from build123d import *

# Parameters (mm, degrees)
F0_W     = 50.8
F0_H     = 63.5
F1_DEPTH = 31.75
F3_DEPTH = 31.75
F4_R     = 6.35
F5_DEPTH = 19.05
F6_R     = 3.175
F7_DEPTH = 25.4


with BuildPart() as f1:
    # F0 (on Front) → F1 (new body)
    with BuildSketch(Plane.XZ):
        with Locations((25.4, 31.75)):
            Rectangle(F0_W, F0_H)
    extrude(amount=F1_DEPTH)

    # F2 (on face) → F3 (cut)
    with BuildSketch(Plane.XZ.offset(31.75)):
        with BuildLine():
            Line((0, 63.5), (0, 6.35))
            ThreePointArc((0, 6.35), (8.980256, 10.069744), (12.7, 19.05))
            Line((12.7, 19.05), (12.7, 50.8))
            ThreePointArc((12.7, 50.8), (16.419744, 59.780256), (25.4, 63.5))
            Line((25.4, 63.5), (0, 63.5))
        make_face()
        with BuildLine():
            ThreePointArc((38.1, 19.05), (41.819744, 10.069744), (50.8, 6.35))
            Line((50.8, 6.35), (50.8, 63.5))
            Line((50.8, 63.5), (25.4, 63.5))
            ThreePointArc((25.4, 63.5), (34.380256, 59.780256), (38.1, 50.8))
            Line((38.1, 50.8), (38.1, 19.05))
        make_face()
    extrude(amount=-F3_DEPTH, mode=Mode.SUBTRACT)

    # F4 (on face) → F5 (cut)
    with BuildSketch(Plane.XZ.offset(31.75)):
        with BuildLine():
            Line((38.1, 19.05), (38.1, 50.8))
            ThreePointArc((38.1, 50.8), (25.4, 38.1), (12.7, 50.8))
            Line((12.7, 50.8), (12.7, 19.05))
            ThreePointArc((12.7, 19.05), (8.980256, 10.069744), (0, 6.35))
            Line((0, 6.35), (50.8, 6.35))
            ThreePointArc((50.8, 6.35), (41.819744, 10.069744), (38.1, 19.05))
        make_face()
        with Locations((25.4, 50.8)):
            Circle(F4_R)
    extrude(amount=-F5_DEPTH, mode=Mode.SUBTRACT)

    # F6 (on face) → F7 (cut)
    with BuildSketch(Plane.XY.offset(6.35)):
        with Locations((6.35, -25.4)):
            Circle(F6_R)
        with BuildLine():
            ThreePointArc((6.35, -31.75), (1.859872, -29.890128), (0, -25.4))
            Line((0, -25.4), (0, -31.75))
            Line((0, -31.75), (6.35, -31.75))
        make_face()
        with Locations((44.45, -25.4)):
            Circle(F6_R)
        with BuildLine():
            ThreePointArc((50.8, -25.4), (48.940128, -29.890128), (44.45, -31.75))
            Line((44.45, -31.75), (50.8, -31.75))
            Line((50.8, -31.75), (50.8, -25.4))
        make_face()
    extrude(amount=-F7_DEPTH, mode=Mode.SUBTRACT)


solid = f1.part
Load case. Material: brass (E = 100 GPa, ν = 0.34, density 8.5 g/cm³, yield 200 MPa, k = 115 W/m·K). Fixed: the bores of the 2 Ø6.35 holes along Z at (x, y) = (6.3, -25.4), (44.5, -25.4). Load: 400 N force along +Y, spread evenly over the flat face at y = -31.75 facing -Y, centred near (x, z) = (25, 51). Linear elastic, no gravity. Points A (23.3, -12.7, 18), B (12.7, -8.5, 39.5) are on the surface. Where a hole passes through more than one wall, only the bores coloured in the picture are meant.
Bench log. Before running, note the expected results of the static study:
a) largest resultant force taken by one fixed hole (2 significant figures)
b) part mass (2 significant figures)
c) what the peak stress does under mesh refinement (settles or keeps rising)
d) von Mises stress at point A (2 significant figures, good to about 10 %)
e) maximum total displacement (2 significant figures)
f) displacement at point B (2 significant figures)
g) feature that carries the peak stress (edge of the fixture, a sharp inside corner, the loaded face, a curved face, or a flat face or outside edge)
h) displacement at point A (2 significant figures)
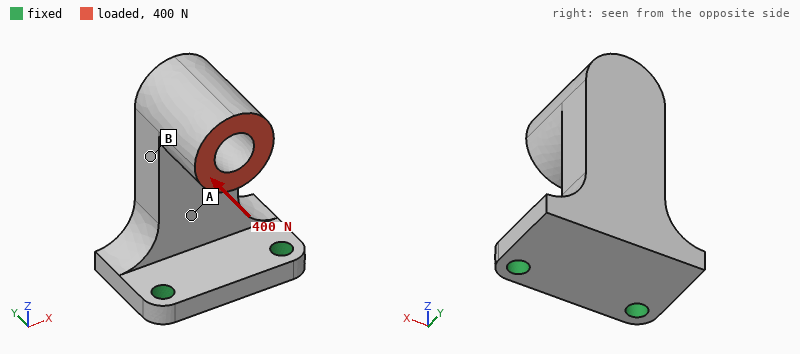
240 N
300 g
keeps rising
19 MPa
0.22 mm
0.12 mm
edge of the fixture
0.047 mm
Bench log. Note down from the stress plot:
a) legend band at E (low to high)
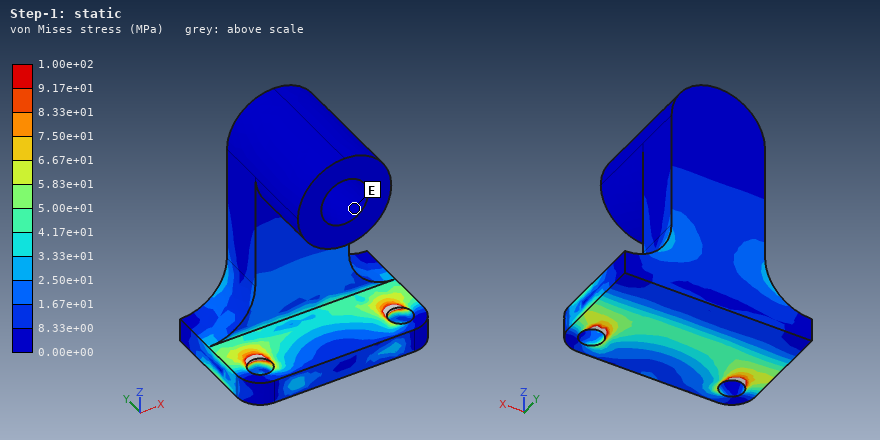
0.00e+00 to 8.33e+00 MPa
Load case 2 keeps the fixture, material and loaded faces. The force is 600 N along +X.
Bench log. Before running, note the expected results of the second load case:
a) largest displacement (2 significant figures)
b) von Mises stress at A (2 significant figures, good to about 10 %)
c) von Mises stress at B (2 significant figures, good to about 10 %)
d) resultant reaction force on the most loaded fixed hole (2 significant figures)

98 µm
31 MPa
18 MPa
830 N
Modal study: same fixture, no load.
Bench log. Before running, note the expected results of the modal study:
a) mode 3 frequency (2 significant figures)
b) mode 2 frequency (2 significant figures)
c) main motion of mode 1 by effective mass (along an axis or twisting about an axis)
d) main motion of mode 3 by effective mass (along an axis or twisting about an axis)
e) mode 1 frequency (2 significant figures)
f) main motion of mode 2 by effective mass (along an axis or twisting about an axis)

2900 Hz
1500 Hz
along Y
along Z
640 Hz
along X
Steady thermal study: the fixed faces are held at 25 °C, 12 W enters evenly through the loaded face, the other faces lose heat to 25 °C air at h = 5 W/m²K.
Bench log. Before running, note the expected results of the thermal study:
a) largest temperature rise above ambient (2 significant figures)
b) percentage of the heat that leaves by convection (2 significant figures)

24 K
4.9 %
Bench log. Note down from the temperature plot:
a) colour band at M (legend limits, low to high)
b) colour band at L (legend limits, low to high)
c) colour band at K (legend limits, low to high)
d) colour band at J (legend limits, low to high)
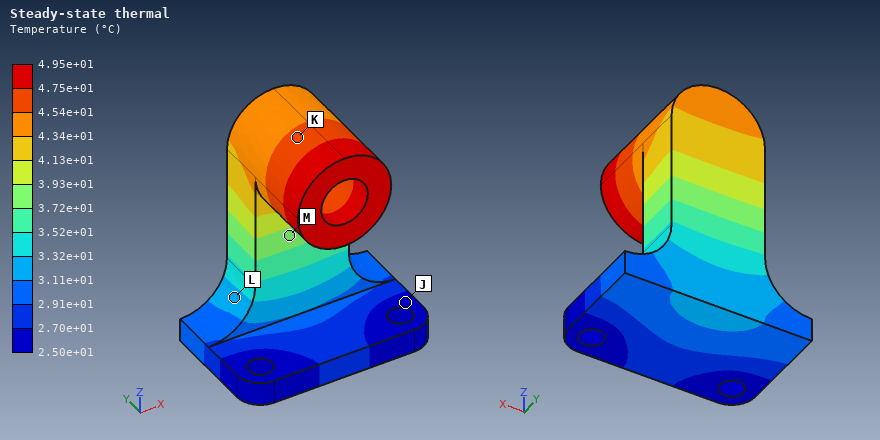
3.72e+01 to 3.93e+01 °C
3.11e+01 to 3.32e+01 °C
4.54e+01 to 4.75e+01 °C
2.50e+01 to 2.70e+01 °C
